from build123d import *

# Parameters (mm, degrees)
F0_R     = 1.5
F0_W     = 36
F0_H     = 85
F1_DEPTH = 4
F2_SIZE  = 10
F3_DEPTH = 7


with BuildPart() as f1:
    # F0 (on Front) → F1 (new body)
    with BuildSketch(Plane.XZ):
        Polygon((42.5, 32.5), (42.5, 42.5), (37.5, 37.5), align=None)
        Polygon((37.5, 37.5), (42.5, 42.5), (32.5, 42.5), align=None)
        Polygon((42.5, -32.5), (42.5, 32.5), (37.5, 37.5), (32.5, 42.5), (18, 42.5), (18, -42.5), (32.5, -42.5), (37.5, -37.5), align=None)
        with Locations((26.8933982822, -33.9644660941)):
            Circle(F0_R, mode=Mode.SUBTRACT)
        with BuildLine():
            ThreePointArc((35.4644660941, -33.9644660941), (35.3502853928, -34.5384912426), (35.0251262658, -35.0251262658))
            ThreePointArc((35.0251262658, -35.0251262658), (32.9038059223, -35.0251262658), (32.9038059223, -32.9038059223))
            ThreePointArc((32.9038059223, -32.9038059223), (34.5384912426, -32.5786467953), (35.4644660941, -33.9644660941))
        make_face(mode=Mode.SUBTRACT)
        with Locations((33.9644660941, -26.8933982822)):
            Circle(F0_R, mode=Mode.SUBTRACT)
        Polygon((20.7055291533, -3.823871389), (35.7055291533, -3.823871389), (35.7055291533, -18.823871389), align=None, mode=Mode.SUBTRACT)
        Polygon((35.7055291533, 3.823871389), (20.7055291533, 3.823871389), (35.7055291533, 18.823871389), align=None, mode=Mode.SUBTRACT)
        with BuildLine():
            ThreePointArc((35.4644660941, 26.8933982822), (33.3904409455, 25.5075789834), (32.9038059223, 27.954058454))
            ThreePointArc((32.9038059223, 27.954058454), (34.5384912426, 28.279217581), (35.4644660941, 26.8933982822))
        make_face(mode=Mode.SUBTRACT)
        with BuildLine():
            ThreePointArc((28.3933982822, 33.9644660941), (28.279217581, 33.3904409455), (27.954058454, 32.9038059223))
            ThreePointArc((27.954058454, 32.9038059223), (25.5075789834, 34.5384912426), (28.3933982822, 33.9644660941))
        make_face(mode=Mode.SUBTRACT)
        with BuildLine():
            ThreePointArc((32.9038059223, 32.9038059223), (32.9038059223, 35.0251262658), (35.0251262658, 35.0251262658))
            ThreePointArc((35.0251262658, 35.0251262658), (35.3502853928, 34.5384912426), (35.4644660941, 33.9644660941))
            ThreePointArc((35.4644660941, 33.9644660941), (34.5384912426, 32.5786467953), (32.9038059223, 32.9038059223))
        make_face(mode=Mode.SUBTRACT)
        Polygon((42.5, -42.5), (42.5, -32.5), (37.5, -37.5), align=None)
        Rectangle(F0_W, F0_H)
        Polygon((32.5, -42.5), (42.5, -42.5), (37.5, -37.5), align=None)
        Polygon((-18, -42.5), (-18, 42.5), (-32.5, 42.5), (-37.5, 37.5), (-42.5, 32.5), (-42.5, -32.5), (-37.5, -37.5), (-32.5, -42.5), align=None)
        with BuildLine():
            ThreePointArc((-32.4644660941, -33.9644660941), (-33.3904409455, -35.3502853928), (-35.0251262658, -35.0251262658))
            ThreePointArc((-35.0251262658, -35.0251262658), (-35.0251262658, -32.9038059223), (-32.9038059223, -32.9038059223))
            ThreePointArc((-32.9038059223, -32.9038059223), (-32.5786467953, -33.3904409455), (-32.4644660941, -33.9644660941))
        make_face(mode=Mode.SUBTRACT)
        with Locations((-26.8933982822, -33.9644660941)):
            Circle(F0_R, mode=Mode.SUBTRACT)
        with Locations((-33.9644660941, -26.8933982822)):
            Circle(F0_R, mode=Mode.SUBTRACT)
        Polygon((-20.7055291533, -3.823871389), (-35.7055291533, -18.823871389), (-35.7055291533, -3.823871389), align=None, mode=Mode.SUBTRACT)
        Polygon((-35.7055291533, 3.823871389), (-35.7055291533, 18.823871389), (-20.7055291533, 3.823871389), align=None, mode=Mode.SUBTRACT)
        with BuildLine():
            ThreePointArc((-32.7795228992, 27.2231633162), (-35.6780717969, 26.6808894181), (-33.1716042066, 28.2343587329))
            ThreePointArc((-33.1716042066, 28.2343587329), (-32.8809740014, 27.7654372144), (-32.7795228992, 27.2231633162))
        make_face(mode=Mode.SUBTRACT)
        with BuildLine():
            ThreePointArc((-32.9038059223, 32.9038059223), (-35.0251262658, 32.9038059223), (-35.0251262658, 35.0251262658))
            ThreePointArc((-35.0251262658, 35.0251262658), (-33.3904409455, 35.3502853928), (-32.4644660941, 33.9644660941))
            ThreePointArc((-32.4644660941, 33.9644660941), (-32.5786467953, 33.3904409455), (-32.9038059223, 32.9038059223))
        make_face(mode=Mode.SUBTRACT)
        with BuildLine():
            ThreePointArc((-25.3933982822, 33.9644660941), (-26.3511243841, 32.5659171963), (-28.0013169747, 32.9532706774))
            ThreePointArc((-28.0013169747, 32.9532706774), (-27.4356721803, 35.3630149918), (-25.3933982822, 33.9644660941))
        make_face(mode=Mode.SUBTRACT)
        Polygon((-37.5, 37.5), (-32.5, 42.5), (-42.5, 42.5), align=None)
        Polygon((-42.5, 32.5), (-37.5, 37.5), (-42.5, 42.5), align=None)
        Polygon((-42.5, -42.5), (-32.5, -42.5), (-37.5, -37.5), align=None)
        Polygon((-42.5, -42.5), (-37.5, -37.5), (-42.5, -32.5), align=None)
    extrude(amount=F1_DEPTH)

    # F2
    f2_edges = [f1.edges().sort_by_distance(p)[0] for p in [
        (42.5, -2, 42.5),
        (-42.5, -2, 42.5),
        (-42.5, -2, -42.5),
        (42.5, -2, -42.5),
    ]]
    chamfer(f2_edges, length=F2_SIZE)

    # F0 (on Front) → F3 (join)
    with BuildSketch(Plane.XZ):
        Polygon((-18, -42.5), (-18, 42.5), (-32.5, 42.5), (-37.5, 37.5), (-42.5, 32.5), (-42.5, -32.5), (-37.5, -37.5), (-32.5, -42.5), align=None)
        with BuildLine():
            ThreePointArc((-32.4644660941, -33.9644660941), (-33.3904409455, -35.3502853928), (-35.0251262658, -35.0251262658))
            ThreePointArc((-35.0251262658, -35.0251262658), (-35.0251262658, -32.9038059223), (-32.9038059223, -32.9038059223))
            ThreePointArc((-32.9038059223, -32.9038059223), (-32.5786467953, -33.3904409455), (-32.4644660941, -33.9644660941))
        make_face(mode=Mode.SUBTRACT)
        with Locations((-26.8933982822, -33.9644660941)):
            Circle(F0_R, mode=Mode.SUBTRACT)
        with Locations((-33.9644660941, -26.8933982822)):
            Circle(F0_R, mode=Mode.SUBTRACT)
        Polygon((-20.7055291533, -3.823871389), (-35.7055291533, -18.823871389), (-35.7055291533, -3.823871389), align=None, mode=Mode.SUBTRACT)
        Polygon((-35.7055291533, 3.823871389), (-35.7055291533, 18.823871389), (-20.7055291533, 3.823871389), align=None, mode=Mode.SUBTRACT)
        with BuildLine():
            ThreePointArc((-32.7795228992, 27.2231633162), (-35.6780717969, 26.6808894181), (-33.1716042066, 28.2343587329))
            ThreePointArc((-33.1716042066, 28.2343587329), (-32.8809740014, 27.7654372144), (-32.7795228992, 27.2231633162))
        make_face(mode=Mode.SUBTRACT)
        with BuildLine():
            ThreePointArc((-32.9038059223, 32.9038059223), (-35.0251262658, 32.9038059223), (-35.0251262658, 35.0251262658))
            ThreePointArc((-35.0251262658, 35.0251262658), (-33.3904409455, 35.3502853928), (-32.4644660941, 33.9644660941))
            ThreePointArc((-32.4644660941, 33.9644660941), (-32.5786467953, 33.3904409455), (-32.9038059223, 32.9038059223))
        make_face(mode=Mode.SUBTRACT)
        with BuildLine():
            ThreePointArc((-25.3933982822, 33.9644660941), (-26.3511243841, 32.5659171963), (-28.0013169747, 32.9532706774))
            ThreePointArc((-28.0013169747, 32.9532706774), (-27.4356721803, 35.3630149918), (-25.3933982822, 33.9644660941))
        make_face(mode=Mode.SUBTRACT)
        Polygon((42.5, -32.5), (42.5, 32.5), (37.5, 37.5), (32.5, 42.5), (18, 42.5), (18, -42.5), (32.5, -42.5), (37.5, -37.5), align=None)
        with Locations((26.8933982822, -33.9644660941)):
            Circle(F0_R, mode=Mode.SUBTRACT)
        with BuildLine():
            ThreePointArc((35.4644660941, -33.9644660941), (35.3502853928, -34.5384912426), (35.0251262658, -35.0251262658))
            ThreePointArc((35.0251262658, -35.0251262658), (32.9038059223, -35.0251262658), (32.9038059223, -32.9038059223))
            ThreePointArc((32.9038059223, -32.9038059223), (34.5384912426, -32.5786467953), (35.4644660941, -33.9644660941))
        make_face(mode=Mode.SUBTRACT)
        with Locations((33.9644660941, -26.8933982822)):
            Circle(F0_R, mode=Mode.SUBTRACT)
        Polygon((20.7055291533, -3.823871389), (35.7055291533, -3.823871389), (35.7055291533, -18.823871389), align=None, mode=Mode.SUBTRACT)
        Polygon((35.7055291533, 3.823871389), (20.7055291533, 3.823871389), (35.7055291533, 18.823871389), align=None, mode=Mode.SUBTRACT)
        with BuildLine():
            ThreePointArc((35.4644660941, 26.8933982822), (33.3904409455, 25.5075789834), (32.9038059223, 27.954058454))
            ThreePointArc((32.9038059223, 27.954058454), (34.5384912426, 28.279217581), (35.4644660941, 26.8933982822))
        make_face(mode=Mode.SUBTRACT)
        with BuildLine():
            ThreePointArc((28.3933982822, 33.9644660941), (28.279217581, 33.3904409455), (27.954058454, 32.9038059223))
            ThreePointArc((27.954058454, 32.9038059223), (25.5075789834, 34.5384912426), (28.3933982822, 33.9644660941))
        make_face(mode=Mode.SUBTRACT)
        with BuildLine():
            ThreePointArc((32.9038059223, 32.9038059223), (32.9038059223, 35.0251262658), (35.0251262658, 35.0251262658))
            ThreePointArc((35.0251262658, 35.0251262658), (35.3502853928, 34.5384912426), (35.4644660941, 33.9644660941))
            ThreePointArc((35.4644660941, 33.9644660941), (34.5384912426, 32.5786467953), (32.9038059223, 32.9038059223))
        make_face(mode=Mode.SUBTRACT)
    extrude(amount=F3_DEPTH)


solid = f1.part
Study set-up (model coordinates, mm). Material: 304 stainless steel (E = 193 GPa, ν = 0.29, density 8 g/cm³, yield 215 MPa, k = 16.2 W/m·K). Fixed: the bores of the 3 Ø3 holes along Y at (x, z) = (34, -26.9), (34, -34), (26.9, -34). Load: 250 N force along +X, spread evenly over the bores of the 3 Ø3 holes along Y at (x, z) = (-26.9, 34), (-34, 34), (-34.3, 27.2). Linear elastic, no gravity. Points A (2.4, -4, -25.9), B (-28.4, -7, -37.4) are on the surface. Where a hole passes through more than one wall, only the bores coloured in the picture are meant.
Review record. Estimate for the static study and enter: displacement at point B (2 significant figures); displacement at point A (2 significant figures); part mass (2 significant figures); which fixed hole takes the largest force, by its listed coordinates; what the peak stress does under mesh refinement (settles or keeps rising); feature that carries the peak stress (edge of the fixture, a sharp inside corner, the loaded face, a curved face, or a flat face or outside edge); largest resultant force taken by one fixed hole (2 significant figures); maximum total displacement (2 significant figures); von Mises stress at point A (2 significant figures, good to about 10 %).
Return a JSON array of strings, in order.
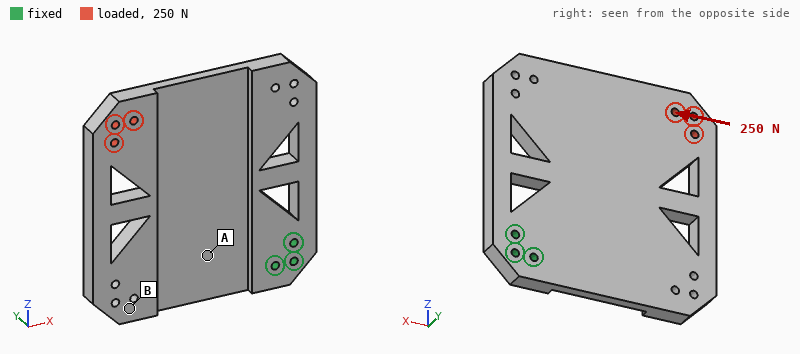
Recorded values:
["11 µm", "4.4 µm", "290 g", "(34, -26.9)", "keeps rising", "edge of the fixture", "1.1 kN", "18 µm", "4.3 MPa"]
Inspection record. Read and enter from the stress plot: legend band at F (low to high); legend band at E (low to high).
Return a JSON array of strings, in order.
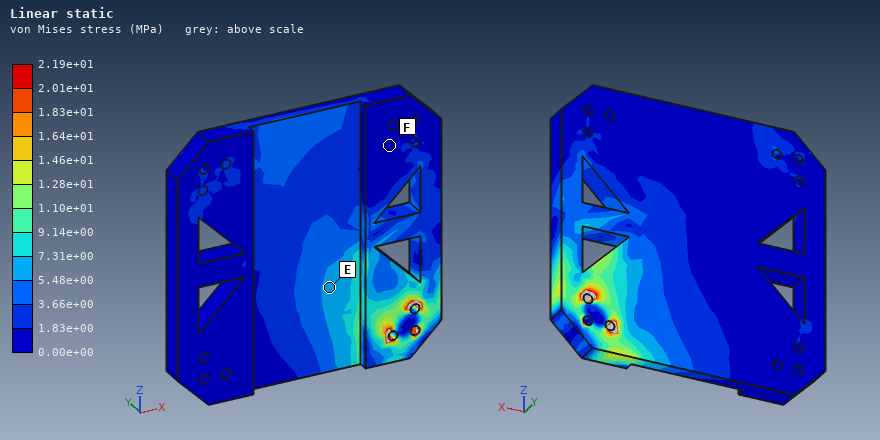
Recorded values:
["0.00e+00 to 1.83e+00 MPa", "5.48e+00 to 7.31e+00 MPa"]
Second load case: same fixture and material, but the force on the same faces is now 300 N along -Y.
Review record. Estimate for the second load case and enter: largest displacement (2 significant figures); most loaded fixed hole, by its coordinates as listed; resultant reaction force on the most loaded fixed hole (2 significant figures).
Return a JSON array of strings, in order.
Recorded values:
["0.64 mm", "(34, -34)", "470 N"]
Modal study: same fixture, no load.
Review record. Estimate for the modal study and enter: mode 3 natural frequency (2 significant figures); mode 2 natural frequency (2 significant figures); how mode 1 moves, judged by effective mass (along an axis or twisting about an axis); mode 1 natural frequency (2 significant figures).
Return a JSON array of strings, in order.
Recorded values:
["1600 Hz", "870 Hz", "along Y", "450 Hz"]
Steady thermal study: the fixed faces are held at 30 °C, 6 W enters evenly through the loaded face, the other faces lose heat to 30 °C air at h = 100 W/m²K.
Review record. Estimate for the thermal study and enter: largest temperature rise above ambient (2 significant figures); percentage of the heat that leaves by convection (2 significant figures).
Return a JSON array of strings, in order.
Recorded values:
["30 K", "99 %"]
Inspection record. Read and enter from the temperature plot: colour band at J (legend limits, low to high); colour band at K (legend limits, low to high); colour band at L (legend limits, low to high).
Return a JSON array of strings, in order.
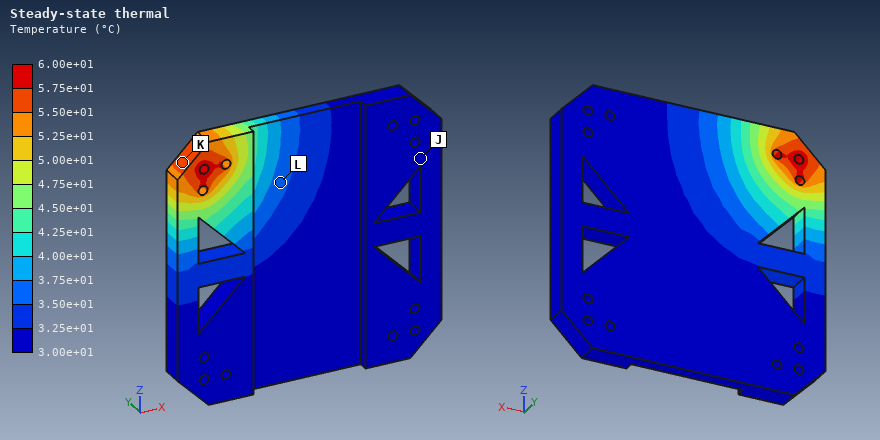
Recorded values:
["3.00e+01 to 3.25e+01 °C", "5.50e+01 to 5.75e+01 °C", "3.50e+01 to 3.75e+01 °C"]
